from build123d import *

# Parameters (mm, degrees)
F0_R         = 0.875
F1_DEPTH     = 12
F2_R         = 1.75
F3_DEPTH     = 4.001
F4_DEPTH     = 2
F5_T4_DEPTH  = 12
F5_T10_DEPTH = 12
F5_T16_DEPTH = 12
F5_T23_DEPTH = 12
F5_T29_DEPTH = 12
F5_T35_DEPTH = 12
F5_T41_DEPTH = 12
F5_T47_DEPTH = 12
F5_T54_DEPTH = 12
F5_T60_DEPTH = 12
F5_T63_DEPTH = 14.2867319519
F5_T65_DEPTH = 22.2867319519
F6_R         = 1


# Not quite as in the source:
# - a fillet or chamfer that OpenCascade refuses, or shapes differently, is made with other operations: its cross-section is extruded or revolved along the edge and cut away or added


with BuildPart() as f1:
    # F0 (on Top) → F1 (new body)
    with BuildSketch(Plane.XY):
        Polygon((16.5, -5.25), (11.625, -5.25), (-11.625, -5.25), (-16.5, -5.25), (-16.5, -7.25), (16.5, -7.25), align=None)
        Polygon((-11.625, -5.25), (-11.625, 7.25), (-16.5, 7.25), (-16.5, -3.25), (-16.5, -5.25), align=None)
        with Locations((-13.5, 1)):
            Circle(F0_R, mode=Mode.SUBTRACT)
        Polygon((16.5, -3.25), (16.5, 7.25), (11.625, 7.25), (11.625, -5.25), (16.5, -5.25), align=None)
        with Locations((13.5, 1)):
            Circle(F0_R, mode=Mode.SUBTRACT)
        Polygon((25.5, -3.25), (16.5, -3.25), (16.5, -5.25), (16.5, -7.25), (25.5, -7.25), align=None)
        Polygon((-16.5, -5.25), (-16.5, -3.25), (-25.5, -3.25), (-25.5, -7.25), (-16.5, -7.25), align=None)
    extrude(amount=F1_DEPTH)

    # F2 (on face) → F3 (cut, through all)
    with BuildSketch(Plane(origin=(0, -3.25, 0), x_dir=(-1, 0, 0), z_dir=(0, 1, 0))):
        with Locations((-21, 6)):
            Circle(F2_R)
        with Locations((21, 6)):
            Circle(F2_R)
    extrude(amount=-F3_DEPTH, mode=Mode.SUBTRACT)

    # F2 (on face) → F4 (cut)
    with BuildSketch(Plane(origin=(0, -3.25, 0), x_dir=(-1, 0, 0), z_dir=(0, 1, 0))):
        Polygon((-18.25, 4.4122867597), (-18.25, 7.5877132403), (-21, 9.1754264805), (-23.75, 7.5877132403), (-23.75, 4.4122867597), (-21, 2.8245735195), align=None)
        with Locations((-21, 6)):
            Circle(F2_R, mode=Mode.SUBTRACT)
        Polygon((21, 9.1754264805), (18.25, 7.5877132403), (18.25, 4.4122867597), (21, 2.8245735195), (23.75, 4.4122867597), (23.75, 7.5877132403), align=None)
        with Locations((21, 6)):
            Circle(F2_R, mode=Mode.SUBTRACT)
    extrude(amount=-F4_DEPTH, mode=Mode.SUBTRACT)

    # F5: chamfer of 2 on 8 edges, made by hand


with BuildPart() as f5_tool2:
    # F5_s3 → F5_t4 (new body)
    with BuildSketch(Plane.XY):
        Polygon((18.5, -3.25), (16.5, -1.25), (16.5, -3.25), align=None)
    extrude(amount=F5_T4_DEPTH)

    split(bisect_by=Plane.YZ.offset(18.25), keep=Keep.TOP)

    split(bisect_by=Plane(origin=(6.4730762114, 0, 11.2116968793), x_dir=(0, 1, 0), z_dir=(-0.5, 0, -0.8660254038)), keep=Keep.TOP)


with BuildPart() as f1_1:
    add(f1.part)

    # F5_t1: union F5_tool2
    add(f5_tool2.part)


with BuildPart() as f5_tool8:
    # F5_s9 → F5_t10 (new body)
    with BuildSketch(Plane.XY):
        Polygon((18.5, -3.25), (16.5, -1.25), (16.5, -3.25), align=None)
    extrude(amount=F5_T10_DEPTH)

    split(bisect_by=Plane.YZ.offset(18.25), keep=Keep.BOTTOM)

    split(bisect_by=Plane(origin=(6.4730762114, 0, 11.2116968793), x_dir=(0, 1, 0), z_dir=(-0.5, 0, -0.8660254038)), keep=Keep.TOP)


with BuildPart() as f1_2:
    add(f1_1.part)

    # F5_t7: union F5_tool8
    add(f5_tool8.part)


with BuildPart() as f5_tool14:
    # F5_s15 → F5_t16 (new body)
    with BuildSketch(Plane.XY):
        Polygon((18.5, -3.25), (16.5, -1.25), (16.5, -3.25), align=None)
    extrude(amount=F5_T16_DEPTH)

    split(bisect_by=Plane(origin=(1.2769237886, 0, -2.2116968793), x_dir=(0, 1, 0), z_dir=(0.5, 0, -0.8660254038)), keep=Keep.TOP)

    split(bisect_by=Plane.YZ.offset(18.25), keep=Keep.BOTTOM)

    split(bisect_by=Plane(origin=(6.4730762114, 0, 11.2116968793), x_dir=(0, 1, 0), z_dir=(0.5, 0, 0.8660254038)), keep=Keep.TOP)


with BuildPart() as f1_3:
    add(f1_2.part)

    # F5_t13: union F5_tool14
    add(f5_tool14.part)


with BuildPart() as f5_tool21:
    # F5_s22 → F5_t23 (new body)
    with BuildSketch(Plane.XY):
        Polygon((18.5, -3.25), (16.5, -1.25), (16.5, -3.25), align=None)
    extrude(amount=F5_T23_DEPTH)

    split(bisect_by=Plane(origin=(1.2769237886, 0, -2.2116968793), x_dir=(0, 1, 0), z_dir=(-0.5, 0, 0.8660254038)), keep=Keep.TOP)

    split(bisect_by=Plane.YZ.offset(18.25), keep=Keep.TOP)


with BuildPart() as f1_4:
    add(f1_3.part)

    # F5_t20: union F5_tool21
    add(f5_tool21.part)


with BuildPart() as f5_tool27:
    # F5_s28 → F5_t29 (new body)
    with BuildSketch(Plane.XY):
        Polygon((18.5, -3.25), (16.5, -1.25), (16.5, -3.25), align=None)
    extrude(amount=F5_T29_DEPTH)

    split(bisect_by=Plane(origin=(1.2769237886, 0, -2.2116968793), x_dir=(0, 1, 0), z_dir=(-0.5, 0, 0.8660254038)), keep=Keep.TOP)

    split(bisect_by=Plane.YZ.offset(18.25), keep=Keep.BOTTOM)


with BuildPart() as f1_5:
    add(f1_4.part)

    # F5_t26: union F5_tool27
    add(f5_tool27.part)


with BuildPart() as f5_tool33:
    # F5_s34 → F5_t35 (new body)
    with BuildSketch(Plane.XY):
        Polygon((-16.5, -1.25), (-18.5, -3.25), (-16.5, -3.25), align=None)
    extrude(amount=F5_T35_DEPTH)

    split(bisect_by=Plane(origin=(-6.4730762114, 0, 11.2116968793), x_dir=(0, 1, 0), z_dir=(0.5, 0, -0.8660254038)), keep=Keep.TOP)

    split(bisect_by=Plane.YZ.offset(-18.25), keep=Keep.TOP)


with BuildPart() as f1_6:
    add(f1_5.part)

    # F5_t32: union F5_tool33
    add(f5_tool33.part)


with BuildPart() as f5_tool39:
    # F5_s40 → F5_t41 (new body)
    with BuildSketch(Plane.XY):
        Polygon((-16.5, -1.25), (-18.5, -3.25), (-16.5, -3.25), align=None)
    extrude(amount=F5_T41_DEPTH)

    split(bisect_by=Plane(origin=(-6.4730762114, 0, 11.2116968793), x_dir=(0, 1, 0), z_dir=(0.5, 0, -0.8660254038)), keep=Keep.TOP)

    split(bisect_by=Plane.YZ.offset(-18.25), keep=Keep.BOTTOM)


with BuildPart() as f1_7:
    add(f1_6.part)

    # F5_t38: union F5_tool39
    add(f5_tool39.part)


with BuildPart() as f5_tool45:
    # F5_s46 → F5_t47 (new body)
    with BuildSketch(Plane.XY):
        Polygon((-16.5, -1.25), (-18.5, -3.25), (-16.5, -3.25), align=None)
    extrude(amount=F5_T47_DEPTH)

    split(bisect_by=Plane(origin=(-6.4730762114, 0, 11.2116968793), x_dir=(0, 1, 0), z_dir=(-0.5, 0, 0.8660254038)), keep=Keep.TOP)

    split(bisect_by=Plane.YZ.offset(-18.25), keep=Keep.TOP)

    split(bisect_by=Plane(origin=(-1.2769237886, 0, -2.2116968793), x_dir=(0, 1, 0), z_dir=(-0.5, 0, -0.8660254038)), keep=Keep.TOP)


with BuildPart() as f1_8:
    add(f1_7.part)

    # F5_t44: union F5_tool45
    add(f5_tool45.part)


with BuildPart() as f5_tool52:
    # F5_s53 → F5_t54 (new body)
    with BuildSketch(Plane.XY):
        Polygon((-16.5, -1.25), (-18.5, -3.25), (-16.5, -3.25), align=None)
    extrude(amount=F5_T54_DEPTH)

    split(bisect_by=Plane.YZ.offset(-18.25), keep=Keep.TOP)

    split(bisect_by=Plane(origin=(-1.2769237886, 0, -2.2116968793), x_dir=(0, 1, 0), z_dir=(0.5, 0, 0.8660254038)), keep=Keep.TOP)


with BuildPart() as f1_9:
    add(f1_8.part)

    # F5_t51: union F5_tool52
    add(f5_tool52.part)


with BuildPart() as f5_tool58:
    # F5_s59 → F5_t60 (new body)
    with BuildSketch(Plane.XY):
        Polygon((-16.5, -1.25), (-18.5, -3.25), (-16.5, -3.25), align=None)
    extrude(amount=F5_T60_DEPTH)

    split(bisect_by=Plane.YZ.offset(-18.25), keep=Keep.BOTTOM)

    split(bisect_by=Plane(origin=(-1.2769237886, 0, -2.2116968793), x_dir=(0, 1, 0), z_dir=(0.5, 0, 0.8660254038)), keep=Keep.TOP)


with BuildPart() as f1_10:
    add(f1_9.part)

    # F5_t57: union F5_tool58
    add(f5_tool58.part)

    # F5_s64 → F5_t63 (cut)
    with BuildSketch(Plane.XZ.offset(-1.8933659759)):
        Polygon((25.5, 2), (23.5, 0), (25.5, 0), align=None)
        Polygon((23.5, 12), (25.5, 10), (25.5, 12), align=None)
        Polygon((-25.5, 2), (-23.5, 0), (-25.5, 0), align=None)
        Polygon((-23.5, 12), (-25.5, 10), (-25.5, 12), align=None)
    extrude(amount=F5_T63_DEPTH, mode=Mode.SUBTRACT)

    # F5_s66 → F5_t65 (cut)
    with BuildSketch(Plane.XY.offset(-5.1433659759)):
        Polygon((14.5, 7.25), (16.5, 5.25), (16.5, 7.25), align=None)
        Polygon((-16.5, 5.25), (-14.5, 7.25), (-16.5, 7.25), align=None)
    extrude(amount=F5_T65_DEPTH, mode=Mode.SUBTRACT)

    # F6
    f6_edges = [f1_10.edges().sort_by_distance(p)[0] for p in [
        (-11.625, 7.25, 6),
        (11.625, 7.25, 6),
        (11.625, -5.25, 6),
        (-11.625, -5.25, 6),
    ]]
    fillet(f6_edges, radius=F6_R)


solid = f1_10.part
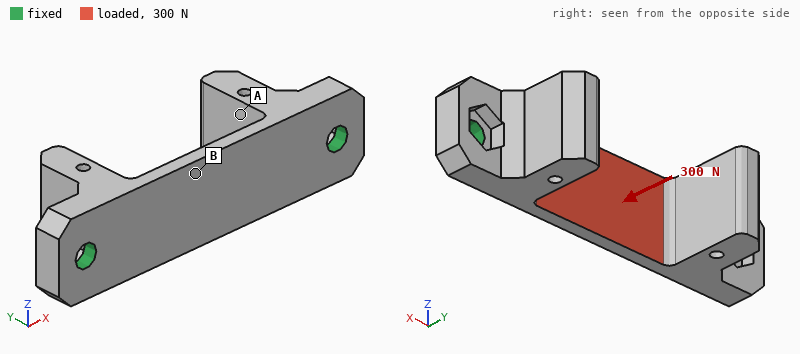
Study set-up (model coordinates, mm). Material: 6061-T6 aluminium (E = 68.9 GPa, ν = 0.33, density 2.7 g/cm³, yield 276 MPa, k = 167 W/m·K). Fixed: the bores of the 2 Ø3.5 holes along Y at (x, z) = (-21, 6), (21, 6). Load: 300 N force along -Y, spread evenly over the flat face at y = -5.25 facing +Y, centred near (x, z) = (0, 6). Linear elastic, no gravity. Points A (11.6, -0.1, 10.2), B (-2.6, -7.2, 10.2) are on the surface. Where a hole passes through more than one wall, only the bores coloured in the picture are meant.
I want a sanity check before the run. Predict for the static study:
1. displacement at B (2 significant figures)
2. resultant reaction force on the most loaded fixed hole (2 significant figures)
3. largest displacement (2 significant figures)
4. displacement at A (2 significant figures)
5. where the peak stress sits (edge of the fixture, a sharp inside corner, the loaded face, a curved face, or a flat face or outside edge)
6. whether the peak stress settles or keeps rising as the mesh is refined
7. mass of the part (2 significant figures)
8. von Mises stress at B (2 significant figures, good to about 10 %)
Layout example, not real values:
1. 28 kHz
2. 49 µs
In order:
1. 66 µm
2. 180 N
3. 71 µm
4. 33 µm
5. edge of the fixture
6. keeps rising
7. 7.8 g
8. 59 MPa
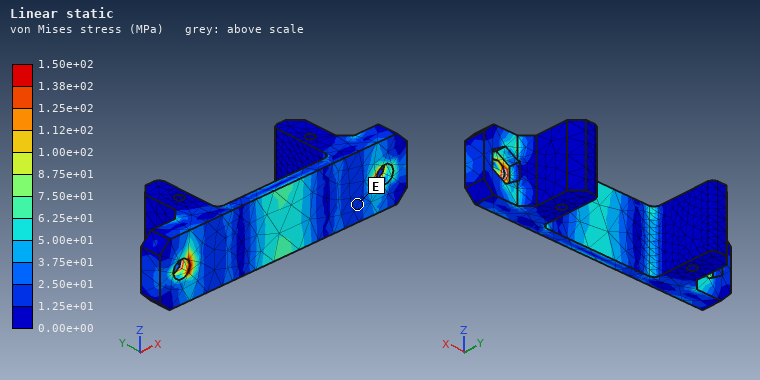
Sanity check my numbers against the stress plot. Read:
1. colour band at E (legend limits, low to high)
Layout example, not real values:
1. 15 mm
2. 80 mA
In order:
1. 1.25e+01 to 2.50e+01 MPa
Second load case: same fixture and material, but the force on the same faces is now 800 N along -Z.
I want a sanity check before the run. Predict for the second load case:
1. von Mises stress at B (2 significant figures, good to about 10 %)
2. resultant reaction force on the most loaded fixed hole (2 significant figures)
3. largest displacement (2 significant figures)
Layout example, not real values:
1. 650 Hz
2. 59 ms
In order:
1. 56 MPa
2. 400 N
3. 35 µm
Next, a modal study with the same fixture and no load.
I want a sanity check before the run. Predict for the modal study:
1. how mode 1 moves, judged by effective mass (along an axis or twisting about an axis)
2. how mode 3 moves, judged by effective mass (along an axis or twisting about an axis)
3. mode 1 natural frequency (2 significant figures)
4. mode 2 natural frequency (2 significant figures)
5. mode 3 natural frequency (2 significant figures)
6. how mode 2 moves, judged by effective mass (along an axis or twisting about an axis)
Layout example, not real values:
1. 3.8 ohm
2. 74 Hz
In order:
1. along Y
2. along Z
3. 6700 Hz
4. 9700 Hz
5. 10 kHz
6. along X
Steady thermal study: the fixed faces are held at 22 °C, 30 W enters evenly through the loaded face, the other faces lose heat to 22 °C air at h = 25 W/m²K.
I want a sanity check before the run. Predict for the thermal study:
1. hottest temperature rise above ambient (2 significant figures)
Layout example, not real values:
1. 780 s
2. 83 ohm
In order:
1. 44 K
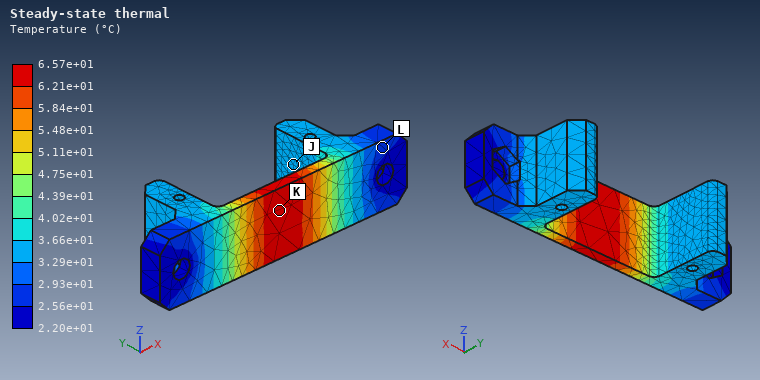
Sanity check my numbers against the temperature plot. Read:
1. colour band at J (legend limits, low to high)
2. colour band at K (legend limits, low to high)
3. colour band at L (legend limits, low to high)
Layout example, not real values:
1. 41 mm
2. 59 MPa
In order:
1. 3.29e+01 to 3.66e+01 °C
2. 6.21e+01 to 6.57e+01 °C
3. 2.56e+01 to 2.93e+01 °C
